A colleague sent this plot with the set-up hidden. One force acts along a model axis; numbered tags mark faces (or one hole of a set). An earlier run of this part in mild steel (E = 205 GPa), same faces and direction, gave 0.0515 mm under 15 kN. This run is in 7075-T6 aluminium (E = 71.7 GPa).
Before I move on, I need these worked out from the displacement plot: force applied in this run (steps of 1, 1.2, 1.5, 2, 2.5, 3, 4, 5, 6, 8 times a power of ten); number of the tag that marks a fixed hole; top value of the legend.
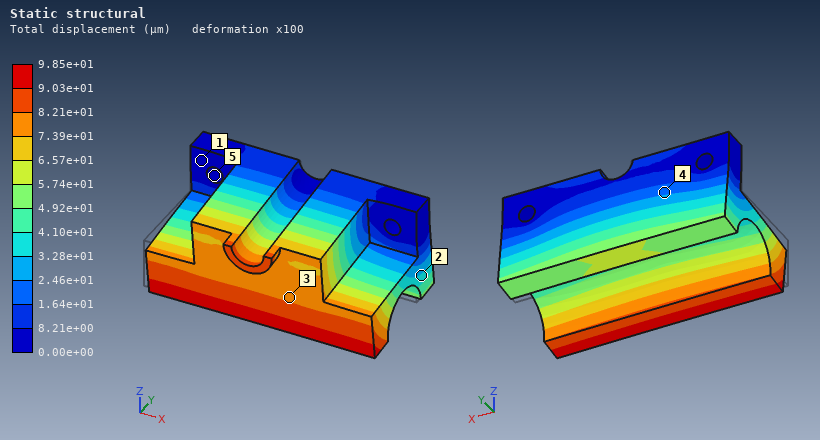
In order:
10 kN
5
9.85e+01 µm
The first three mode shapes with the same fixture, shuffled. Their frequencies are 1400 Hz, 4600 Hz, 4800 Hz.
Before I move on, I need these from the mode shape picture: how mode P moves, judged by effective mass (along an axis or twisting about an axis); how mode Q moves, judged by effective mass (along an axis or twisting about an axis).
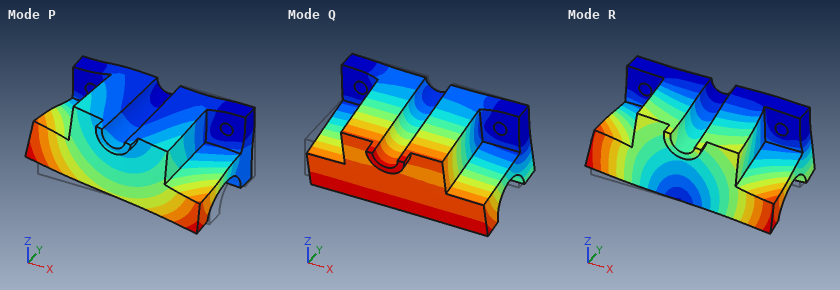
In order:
along X
along Z
